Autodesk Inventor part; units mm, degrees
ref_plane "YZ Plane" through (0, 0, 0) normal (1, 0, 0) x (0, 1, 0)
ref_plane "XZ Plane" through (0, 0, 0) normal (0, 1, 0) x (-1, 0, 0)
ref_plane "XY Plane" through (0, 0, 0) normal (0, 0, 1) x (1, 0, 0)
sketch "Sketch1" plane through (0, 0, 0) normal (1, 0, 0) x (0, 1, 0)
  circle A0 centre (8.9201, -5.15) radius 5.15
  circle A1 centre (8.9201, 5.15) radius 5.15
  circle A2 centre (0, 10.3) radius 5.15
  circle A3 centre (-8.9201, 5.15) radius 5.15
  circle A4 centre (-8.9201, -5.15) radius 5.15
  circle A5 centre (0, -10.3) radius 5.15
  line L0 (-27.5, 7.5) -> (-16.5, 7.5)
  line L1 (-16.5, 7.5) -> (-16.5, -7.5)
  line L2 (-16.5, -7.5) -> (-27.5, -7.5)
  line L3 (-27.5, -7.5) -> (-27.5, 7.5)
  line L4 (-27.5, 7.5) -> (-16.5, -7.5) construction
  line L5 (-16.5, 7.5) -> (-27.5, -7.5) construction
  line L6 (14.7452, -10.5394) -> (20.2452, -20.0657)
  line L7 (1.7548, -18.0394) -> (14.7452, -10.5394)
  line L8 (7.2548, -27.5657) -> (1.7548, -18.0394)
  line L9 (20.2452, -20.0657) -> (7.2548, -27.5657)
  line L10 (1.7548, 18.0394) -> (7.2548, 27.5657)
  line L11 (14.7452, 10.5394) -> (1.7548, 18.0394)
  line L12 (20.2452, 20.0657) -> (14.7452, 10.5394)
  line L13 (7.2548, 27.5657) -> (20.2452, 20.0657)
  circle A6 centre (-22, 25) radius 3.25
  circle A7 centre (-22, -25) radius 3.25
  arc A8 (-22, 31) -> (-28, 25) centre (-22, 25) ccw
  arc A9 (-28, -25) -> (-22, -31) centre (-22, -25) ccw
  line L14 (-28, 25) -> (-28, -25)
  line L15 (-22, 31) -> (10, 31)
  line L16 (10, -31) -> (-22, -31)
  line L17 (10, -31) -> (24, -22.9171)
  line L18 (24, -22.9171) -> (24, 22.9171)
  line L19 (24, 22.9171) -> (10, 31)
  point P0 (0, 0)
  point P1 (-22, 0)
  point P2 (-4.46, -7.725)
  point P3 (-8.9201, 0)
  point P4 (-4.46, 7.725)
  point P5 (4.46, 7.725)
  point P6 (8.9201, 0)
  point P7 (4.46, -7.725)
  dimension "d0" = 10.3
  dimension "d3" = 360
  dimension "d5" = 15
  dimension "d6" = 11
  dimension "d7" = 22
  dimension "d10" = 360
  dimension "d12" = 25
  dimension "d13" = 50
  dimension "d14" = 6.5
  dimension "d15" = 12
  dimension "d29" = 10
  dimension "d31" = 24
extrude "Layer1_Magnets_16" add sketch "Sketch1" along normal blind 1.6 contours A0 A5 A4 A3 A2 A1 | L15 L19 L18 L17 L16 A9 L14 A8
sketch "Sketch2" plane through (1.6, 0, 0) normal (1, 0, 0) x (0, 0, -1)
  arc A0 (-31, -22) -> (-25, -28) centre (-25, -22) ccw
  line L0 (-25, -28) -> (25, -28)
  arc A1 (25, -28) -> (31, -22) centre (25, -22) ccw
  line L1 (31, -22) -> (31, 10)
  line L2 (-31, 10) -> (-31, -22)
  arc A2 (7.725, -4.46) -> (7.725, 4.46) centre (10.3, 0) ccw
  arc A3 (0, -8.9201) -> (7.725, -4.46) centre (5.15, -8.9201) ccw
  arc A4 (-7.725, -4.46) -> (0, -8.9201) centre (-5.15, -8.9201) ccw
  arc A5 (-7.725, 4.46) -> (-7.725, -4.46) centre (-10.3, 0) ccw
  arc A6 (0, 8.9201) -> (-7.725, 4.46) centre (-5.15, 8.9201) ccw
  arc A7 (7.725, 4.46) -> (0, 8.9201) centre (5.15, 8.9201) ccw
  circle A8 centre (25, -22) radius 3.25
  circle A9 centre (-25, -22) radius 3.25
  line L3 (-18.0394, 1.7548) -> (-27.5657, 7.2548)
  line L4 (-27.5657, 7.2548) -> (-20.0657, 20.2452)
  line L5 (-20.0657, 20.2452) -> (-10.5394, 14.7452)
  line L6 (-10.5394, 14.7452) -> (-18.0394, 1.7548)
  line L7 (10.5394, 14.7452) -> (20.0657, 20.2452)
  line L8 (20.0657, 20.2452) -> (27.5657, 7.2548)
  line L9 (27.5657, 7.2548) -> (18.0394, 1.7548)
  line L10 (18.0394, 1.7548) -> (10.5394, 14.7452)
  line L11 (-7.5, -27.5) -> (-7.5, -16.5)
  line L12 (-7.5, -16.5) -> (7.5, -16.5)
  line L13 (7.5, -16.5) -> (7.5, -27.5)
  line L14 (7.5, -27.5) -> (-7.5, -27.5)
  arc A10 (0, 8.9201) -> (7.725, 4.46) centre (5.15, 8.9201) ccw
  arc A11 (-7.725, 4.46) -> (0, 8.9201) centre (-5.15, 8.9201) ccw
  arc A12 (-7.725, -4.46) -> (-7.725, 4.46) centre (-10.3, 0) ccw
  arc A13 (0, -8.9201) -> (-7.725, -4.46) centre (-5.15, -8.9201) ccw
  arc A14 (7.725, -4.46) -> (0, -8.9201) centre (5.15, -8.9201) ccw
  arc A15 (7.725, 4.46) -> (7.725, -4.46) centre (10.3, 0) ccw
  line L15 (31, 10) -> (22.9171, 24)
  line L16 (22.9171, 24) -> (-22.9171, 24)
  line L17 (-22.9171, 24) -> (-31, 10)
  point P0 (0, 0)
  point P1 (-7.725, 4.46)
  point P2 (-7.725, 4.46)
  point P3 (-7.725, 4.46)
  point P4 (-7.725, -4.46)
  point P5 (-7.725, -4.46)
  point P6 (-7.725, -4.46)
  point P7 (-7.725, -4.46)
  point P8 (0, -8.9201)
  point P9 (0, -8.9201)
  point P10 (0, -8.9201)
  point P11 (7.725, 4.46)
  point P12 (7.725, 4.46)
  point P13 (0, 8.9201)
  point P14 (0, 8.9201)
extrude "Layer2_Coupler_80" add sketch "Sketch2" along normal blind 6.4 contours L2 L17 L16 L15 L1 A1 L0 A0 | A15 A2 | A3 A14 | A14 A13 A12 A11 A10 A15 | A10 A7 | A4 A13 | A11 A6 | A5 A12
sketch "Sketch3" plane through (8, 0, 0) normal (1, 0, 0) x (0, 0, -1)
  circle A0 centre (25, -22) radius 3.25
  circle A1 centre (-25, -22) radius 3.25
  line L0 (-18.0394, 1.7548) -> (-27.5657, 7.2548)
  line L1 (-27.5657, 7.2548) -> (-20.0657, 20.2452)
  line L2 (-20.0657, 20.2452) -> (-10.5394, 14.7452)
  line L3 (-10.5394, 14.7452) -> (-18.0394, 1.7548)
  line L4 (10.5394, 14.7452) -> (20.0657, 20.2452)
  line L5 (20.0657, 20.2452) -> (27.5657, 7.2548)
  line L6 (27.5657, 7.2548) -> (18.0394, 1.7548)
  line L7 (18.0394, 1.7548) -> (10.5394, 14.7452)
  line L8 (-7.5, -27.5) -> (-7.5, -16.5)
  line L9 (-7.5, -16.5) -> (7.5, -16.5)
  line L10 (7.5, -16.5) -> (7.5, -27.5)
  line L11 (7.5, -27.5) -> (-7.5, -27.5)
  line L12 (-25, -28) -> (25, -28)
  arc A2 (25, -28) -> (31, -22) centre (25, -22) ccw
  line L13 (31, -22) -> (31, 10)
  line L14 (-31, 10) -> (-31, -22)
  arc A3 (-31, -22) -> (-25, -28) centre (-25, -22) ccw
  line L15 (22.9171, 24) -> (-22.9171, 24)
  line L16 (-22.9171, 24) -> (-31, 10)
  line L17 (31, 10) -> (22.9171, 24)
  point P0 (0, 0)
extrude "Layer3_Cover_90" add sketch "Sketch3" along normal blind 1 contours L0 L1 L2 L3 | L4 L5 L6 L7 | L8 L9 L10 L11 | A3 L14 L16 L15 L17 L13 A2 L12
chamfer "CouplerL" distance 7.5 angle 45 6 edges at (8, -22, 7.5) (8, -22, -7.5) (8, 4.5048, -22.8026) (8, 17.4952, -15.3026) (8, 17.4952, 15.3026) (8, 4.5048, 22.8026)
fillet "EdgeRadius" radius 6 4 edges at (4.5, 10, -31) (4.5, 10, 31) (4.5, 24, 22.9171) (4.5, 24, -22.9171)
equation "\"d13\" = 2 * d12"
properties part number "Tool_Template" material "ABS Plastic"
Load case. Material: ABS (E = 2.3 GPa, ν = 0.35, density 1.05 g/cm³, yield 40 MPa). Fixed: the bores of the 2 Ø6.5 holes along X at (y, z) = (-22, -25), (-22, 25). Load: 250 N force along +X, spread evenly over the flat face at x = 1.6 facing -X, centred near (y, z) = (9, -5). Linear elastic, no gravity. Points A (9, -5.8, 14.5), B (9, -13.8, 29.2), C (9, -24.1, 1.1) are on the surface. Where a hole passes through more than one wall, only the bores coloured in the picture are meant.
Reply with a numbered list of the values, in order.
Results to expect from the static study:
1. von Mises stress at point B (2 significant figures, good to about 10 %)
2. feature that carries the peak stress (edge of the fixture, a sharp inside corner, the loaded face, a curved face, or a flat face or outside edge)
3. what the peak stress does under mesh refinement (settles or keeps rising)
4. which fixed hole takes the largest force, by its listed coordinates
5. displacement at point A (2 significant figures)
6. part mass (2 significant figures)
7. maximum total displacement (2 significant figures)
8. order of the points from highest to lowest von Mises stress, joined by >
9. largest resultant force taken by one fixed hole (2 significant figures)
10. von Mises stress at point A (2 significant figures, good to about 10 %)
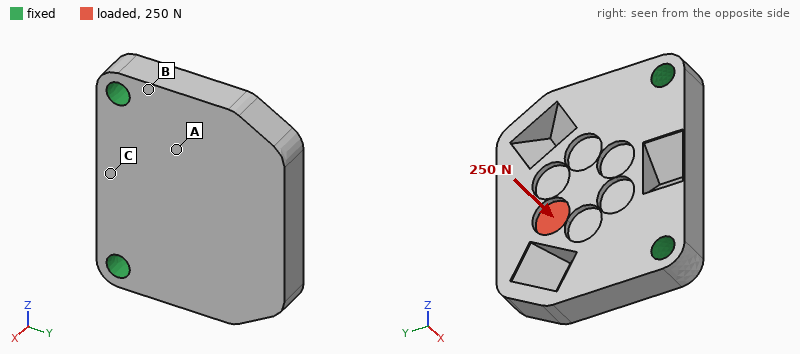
1. 8.7 MPa
2. edge of the fixture
3. keeps rising
4. (-22, -25)
5. 0.19 mm
6. 26 g
7. 0.84 mm
8. B > A > C
9. 150 N
10. 4.8 MPa
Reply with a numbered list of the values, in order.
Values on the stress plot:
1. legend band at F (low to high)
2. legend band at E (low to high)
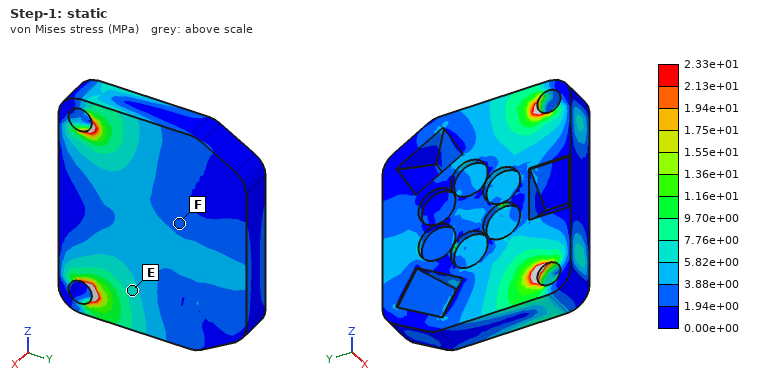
1. 1.94e+00 to 3.88e+00 MPa
2. 5.82e+00 to 7.76e+00 MPa
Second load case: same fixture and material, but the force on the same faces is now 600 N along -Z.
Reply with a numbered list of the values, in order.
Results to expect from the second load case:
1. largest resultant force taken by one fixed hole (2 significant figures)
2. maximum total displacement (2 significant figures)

1. 460 N
2. 0.16 mm
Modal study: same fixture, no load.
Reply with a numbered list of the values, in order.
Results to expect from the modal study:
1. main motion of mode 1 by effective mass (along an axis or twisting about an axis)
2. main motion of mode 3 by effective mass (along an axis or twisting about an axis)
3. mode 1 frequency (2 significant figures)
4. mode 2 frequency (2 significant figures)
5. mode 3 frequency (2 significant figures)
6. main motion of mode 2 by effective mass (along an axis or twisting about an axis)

1. along X
2. along Z
3. 930 Hz
4. 2100 Hz
5. 4000 Hz
6. twisting about Y
